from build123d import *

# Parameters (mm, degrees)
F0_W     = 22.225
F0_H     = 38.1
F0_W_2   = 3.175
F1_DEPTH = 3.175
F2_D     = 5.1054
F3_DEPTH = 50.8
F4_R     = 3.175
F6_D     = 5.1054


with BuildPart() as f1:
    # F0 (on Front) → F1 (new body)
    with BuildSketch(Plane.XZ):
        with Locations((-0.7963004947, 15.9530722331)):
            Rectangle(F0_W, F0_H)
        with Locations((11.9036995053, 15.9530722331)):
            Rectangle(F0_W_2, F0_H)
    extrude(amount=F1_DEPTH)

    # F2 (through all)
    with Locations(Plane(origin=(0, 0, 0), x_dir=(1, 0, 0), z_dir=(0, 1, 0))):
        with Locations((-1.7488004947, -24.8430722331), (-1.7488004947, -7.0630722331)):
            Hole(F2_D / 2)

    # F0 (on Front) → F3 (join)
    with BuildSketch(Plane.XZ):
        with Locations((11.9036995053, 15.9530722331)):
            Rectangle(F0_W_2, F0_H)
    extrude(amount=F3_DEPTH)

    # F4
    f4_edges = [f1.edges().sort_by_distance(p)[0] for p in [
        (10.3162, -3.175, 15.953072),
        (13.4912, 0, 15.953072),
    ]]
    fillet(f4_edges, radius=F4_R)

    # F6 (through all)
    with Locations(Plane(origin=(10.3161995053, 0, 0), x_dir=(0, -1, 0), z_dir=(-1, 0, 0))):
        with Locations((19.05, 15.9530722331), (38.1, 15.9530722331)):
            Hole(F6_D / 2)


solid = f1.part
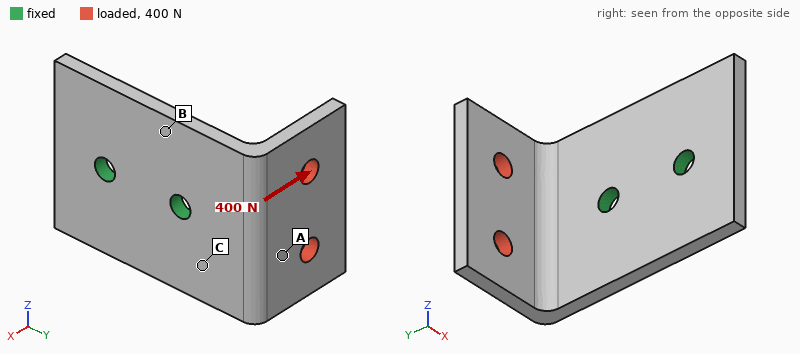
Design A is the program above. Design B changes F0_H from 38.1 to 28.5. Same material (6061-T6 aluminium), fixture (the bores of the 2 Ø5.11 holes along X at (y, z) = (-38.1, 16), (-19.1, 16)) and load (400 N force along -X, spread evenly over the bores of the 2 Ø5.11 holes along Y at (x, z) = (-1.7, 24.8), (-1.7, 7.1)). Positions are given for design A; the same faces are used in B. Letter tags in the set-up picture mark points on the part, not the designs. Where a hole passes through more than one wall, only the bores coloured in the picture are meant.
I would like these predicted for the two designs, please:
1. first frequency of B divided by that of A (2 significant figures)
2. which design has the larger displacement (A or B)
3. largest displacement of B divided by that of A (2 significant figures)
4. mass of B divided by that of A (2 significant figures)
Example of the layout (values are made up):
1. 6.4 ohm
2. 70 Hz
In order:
1. 1.0
2. B
3. 1.2
4. 0.74
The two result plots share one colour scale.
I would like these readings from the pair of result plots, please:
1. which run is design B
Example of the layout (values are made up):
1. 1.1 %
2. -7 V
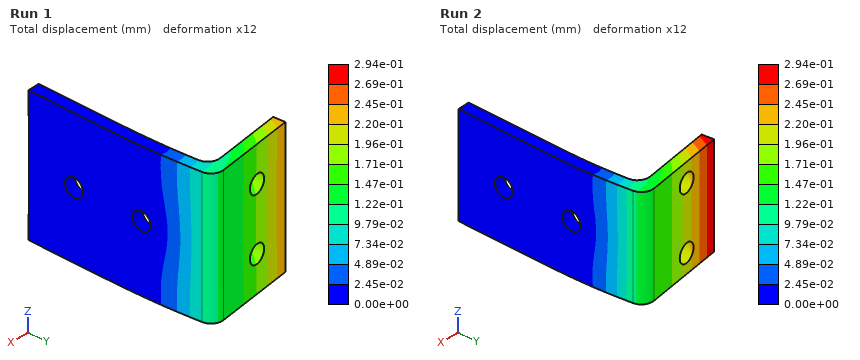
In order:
1. Run 2
